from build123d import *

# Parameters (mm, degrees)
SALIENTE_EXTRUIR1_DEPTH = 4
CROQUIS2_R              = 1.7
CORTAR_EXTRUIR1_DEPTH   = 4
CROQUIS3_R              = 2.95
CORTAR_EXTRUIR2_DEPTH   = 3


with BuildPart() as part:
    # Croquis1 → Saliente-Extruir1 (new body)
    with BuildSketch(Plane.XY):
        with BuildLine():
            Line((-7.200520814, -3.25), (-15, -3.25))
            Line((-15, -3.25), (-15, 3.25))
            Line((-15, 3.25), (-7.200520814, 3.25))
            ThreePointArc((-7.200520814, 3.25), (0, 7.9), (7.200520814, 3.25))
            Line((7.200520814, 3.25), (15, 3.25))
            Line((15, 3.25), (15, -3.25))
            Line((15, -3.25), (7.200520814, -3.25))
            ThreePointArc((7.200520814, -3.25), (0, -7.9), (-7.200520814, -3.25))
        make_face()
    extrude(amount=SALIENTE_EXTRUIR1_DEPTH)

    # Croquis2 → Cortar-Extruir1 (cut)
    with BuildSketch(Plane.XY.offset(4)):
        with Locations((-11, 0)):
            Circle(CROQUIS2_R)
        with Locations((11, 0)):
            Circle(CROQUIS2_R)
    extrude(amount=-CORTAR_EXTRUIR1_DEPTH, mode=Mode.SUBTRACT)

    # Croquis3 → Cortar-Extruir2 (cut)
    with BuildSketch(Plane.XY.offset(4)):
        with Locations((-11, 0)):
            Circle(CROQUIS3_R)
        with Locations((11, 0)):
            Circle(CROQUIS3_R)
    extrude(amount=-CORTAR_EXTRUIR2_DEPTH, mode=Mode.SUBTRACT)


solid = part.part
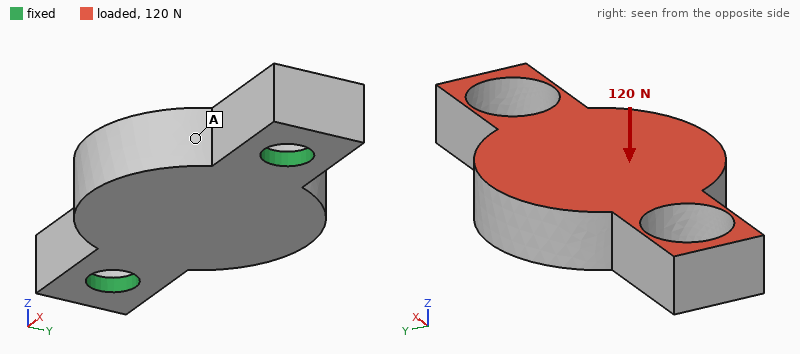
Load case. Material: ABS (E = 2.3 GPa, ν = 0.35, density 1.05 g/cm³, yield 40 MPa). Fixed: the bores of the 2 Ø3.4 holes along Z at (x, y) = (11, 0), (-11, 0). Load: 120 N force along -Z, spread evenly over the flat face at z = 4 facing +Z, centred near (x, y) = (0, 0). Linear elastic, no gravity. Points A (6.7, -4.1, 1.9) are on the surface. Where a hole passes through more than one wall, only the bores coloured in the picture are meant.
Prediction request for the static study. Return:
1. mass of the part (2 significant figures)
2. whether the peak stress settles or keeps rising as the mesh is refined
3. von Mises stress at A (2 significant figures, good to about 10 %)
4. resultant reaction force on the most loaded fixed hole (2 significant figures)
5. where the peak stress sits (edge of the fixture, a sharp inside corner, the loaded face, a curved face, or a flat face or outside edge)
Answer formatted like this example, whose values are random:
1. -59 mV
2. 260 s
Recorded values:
1. 1.0 g
2. keeps rising
3. 6.0 MPa
4. 80 N
5. edge of the fixture
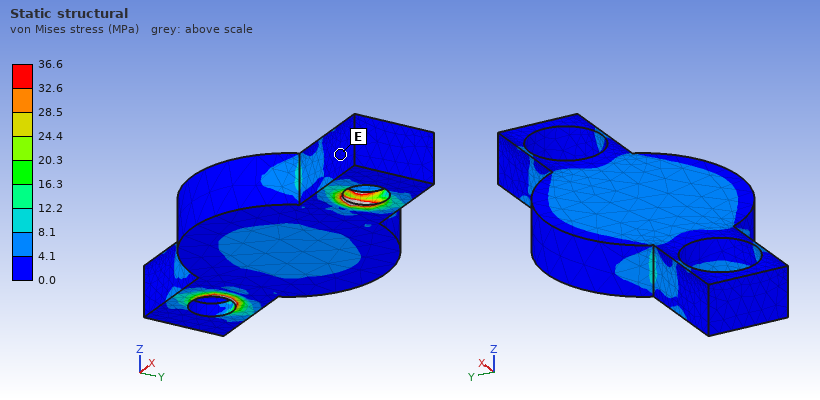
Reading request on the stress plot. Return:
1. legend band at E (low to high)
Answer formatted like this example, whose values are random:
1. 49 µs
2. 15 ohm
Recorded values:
1. 0.0 to 4.1 MPa
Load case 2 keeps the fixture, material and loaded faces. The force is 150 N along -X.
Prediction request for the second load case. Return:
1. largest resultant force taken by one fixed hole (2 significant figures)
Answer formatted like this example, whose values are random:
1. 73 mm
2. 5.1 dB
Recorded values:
1. 79 N
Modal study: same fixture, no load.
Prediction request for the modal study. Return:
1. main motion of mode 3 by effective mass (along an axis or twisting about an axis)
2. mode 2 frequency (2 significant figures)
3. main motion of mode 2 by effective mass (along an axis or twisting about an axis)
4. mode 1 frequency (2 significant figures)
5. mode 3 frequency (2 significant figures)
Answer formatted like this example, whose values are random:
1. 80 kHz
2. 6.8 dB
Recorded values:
1. along Y
2. 6200 Hz
3. along Z
4. 3800 Hz
5. 10 kHz
